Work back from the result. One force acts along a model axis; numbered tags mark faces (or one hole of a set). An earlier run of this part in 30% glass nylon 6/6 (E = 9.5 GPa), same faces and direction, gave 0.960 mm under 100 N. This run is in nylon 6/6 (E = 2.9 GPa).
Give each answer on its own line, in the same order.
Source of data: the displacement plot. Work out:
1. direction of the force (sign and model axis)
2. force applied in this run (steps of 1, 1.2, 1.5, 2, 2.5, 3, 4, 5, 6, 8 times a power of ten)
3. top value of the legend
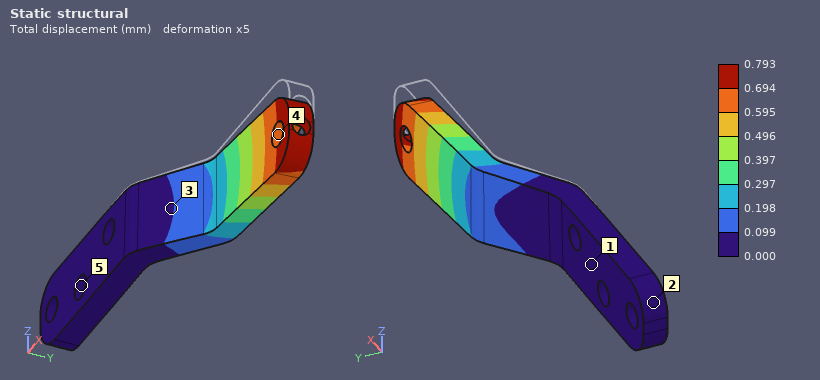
-Z
25 N
0.793 mm
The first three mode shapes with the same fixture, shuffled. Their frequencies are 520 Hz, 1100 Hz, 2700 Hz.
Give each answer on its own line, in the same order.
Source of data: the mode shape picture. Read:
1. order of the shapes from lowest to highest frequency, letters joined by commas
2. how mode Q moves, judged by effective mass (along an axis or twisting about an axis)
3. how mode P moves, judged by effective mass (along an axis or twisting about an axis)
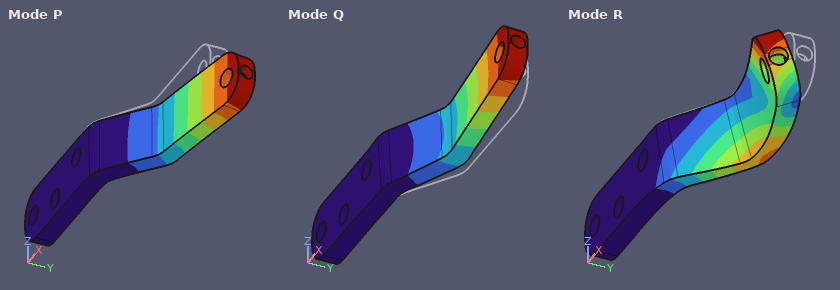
P, Q, R
along Z
along Y
